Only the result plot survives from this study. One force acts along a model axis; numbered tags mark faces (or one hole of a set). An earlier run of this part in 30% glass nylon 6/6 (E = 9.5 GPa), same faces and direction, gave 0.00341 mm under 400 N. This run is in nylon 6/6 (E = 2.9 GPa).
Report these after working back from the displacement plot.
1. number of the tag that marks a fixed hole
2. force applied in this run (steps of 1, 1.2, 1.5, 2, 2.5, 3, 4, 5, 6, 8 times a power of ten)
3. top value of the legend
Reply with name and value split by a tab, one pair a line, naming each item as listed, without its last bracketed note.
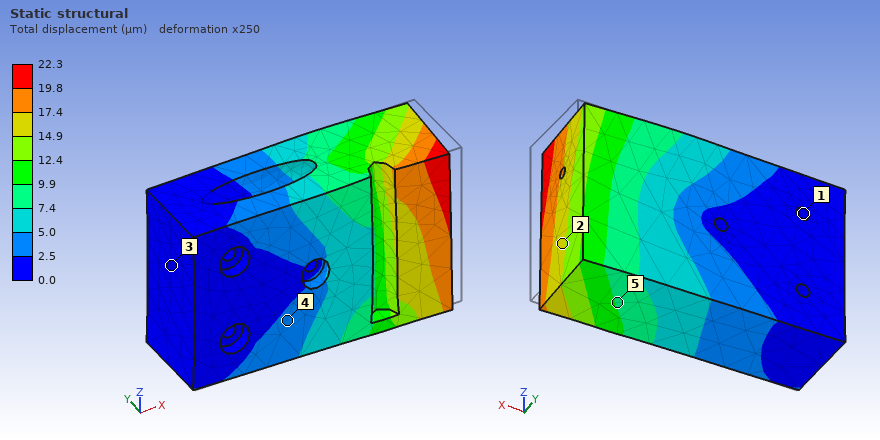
number of the tag that marks a fixed hole	1
force applied in this run	800 N
top value of the legend	22.3 µm
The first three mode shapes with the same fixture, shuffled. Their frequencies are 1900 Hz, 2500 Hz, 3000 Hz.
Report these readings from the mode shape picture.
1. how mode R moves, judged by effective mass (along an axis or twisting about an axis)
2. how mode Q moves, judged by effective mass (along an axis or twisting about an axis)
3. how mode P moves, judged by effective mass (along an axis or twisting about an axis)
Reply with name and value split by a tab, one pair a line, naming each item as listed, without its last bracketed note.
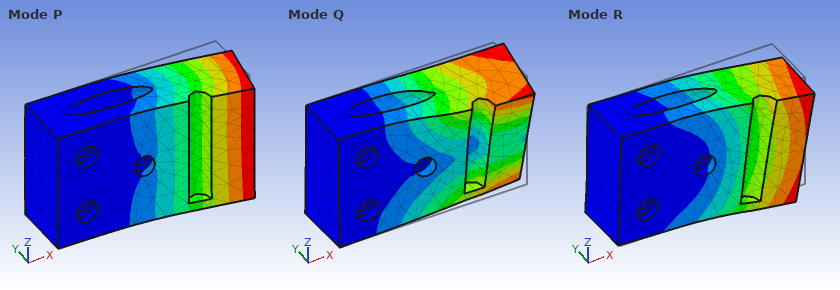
how mode R moves, judged by effective mass	along Z
how mode Q moves, judged by effective mass	twisting about X
how mode P moves, judged by effective mass	along Y
